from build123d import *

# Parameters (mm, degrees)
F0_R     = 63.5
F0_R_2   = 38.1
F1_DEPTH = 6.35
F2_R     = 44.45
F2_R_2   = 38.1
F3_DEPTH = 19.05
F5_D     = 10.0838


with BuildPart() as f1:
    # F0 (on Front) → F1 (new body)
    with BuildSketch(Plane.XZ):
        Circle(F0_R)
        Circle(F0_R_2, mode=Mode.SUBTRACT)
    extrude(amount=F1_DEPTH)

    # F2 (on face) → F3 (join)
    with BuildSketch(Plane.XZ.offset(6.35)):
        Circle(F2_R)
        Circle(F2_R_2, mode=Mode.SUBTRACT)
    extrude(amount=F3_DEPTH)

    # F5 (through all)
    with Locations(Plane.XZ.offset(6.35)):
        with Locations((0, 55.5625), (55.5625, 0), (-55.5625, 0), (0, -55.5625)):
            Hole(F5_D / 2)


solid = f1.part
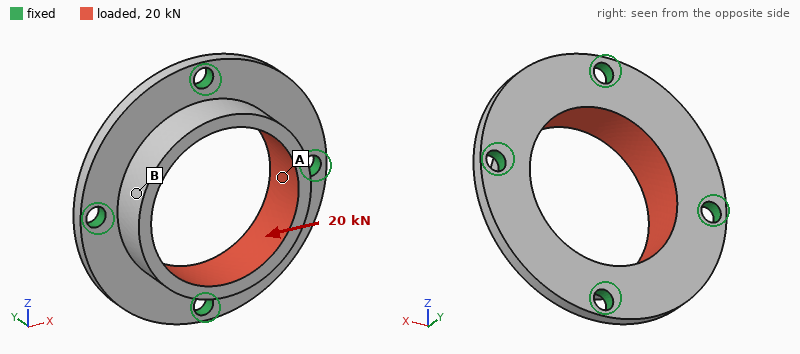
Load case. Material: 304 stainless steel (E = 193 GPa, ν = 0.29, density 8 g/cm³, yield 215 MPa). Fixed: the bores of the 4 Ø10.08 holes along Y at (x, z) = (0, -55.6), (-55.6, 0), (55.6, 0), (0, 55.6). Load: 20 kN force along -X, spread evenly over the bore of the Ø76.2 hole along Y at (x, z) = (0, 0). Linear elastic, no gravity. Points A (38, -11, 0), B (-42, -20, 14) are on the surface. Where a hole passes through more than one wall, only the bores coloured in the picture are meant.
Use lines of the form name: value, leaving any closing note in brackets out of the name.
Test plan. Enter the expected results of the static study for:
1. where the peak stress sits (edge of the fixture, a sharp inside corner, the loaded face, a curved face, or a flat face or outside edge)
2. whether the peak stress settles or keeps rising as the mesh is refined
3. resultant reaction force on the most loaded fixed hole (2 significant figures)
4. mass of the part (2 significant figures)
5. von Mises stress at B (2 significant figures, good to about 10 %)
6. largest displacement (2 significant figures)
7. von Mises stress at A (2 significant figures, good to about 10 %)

where the peak stress sits: edge of the fixture
whether the peak stress settles or keeps rising as the mesh is refined: keeps rising
resultant reaction force on the most loaded fixed hole: 5.9 kN
mass of the part: 650 g
von Mises stress at B: 14 MPa
largest displacement: 14 µm
von Mises stress at A: 29 MPa
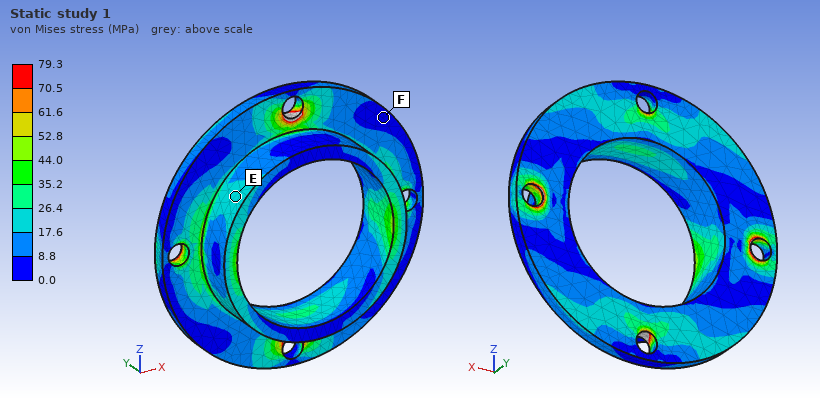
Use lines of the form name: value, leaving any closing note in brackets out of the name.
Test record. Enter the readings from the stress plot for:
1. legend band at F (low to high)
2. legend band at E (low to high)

legend band at F: 0.0 to 8.8 MPa
legend band at E: 17.6 to 26.4 MPa
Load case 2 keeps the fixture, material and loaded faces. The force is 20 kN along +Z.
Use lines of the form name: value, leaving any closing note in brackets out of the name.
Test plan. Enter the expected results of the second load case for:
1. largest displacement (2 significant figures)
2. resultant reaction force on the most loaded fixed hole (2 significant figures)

largest displacement: 14 µm
resultant reaction force on the most loaded fixed hole: 5.9 kN
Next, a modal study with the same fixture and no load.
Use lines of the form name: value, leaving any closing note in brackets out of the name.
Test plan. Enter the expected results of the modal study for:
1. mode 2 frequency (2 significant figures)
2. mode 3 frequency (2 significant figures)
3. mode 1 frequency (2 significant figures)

mode 2 frequency: 6000 Hz
mode 3 frequency: 6000 Hz
mode 1 frequency: 4900 Hz
